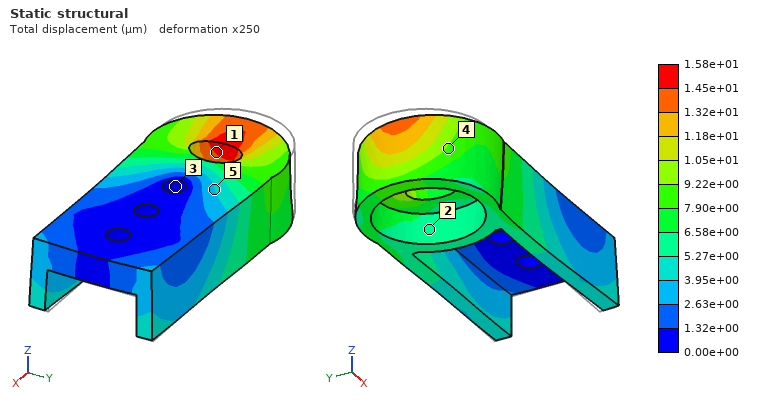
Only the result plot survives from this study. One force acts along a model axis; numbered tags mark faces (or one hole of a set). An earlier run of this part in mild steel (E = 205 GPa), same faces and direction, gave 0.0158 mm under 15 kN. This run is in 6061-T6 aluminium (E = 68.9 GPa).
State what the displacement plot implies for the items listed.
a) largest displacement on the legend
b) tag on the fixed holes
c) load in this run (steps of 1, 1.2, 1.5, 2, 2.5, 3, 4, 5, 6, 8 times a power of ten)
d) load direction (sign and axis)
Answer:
1.58e+01 µm
3
5 kN
+X
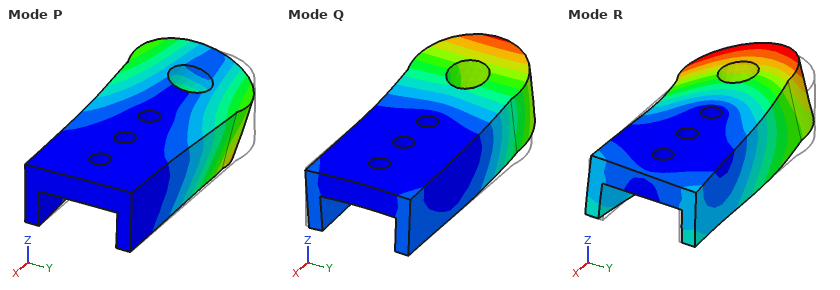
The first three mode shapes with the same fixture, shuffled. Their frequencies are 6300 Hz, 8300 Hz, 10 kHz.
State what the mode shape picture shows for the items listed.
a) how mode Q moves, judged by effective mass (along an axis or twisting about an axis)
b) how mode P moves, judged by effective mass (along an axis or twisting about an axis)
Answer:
along Z
along Y
